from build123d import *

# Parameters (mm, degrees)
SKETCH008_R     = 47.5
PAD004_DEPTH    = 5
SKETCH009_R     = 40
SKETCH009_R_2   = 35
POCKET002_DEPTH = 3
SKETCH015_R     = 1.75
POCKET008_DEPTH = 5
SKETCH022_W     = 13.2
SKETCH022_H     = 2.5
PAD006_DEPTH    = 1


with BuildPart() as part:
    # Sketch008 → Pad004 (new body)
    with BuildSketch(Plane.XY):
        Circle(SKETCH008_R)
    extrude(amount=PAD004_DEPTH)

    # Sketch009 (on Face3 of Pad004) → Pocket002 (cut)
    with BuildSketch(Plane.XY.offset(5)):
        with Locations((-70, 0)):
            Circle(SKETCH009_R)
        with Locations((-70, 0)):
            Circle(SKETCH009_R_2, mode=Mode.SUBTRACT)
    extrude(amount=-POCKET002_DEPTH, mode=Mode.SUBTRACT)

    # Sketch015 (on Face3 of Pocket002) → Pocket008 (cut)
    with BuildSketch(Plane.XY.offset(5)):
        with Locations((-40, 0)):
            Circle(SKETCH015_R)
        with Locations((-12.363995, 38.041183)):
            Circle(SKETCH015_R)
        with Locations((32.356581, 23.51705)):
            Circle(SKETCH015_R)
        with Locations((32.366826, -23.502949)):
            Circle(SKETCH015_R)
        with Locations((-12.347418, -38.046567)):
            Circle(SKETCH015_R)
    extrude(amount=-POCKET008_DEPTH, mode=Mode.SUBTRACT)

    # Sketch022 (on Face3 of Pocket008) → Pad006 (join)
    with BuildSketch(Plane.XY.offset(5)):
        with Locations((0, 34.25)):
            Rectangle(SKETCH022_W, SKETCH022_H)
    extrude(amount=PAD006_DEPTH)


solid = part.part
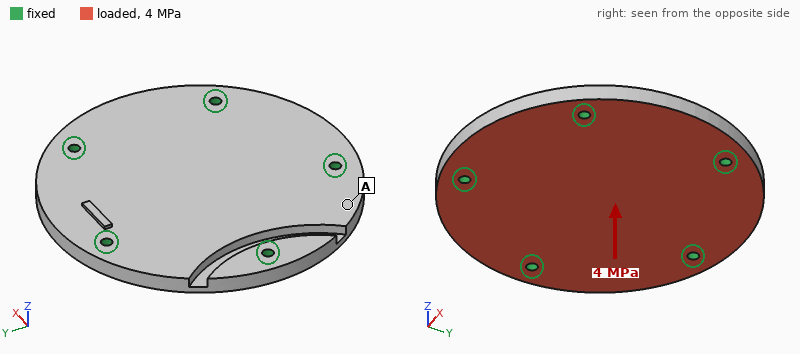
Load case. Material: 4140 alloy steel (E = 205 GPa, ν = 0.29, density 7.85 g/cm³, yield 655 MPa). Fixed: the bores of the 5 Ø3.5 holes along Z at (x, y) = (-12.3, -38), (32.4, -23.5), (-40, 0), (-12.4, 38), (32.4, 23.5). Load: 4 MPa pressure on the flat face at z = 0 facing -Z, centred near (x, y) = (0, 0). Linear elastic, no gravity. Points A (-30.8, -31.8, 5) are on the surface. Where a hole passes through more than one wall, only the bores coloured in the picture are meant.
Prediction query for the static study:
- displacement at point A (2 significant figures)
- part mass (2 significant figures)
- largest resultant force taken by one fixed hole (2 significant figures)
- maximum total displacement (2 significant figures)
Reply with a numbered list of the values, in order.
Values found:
1. 0.031 mm
2. 270 g
3. 5.8 kN
4. 0.12 mm
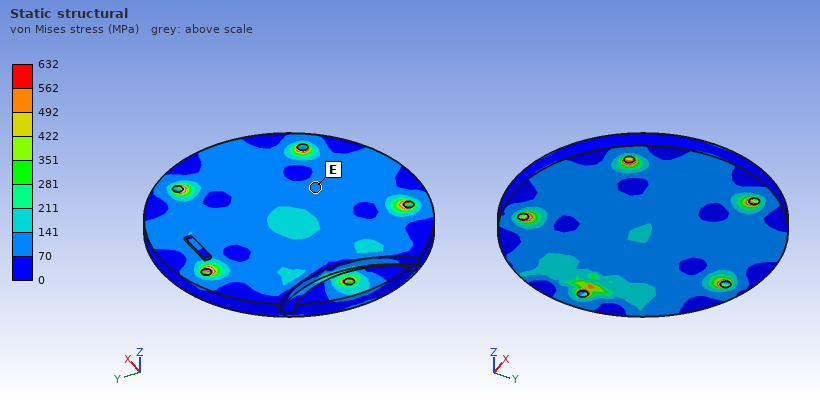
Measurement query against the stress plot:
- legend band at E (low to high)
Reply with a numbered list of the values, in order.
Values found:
1. 70 to 141 MPa
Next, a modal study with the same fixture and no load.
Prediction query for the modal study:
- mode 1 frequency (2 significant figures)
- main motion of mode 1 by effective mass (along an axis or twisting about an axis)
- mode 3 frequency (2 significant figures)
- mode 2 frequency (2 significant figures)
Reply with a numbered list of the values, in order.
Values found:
1. 5600 Hz
2. along Z
3. 8700 Hz
4. 8700 Hz
